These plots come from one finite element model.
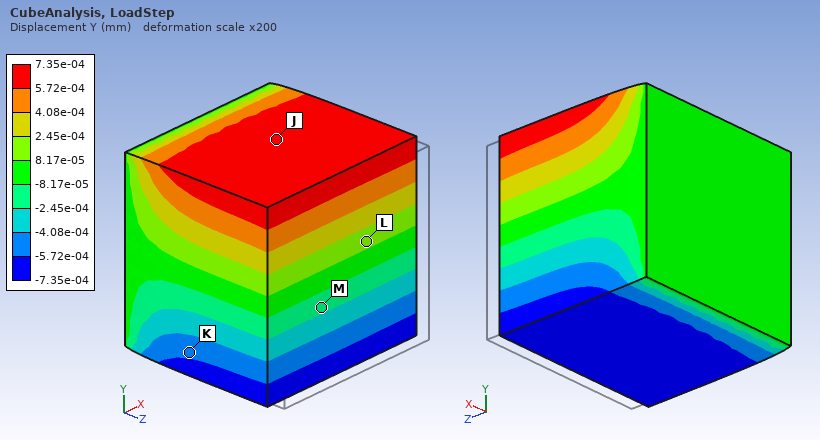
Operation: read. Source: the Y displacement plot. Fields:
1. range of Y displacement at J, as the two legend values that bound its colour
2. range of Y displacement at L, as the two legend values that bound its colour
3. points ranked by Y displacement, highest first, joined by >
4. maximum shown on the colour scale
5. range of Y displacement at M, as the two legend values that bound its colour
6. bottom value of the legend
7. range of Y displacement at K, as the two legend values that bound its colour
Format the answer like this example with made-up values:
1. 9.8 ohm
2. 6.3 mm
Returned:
1. 5.72e-04 to 7.35e-04 mm
2. 8.17e-05 to 2.45e-04 mm
3. J > L > M > K
4. 7.35e-04 mm
5. -2.45e-04 to -8.17e-05 mm
6. -7.35e-04 mm
7. -5.72e-04 to -4.08e-04 mm
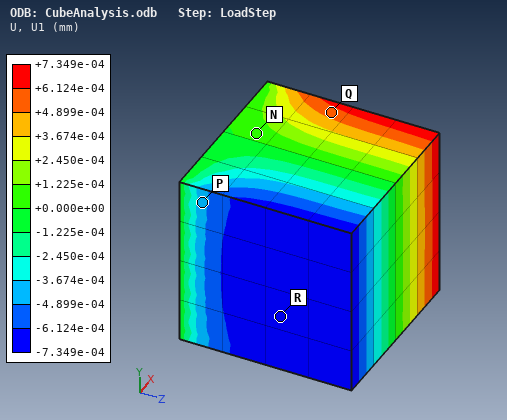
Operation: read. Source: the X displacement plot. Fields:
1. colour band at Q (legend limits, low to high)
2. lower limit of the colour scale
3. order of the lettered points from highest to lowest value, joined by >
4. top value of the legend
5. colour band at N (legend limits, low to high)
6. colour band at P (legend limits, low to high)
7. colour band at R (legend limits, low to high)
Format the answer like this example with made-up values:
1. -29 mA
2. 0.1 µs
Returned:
1. +4.899e-04 to +6.124e-04 mm
2. -7.349e-04 mm
3. Q > N > P > R
4. +7.349e-04 mm
5. +0.000e+00 to +1.225e-04 mm
6. -4.899e-04 to -3.674e-04 mm
7. -7.349e-04 to -6.124e-04 mm
